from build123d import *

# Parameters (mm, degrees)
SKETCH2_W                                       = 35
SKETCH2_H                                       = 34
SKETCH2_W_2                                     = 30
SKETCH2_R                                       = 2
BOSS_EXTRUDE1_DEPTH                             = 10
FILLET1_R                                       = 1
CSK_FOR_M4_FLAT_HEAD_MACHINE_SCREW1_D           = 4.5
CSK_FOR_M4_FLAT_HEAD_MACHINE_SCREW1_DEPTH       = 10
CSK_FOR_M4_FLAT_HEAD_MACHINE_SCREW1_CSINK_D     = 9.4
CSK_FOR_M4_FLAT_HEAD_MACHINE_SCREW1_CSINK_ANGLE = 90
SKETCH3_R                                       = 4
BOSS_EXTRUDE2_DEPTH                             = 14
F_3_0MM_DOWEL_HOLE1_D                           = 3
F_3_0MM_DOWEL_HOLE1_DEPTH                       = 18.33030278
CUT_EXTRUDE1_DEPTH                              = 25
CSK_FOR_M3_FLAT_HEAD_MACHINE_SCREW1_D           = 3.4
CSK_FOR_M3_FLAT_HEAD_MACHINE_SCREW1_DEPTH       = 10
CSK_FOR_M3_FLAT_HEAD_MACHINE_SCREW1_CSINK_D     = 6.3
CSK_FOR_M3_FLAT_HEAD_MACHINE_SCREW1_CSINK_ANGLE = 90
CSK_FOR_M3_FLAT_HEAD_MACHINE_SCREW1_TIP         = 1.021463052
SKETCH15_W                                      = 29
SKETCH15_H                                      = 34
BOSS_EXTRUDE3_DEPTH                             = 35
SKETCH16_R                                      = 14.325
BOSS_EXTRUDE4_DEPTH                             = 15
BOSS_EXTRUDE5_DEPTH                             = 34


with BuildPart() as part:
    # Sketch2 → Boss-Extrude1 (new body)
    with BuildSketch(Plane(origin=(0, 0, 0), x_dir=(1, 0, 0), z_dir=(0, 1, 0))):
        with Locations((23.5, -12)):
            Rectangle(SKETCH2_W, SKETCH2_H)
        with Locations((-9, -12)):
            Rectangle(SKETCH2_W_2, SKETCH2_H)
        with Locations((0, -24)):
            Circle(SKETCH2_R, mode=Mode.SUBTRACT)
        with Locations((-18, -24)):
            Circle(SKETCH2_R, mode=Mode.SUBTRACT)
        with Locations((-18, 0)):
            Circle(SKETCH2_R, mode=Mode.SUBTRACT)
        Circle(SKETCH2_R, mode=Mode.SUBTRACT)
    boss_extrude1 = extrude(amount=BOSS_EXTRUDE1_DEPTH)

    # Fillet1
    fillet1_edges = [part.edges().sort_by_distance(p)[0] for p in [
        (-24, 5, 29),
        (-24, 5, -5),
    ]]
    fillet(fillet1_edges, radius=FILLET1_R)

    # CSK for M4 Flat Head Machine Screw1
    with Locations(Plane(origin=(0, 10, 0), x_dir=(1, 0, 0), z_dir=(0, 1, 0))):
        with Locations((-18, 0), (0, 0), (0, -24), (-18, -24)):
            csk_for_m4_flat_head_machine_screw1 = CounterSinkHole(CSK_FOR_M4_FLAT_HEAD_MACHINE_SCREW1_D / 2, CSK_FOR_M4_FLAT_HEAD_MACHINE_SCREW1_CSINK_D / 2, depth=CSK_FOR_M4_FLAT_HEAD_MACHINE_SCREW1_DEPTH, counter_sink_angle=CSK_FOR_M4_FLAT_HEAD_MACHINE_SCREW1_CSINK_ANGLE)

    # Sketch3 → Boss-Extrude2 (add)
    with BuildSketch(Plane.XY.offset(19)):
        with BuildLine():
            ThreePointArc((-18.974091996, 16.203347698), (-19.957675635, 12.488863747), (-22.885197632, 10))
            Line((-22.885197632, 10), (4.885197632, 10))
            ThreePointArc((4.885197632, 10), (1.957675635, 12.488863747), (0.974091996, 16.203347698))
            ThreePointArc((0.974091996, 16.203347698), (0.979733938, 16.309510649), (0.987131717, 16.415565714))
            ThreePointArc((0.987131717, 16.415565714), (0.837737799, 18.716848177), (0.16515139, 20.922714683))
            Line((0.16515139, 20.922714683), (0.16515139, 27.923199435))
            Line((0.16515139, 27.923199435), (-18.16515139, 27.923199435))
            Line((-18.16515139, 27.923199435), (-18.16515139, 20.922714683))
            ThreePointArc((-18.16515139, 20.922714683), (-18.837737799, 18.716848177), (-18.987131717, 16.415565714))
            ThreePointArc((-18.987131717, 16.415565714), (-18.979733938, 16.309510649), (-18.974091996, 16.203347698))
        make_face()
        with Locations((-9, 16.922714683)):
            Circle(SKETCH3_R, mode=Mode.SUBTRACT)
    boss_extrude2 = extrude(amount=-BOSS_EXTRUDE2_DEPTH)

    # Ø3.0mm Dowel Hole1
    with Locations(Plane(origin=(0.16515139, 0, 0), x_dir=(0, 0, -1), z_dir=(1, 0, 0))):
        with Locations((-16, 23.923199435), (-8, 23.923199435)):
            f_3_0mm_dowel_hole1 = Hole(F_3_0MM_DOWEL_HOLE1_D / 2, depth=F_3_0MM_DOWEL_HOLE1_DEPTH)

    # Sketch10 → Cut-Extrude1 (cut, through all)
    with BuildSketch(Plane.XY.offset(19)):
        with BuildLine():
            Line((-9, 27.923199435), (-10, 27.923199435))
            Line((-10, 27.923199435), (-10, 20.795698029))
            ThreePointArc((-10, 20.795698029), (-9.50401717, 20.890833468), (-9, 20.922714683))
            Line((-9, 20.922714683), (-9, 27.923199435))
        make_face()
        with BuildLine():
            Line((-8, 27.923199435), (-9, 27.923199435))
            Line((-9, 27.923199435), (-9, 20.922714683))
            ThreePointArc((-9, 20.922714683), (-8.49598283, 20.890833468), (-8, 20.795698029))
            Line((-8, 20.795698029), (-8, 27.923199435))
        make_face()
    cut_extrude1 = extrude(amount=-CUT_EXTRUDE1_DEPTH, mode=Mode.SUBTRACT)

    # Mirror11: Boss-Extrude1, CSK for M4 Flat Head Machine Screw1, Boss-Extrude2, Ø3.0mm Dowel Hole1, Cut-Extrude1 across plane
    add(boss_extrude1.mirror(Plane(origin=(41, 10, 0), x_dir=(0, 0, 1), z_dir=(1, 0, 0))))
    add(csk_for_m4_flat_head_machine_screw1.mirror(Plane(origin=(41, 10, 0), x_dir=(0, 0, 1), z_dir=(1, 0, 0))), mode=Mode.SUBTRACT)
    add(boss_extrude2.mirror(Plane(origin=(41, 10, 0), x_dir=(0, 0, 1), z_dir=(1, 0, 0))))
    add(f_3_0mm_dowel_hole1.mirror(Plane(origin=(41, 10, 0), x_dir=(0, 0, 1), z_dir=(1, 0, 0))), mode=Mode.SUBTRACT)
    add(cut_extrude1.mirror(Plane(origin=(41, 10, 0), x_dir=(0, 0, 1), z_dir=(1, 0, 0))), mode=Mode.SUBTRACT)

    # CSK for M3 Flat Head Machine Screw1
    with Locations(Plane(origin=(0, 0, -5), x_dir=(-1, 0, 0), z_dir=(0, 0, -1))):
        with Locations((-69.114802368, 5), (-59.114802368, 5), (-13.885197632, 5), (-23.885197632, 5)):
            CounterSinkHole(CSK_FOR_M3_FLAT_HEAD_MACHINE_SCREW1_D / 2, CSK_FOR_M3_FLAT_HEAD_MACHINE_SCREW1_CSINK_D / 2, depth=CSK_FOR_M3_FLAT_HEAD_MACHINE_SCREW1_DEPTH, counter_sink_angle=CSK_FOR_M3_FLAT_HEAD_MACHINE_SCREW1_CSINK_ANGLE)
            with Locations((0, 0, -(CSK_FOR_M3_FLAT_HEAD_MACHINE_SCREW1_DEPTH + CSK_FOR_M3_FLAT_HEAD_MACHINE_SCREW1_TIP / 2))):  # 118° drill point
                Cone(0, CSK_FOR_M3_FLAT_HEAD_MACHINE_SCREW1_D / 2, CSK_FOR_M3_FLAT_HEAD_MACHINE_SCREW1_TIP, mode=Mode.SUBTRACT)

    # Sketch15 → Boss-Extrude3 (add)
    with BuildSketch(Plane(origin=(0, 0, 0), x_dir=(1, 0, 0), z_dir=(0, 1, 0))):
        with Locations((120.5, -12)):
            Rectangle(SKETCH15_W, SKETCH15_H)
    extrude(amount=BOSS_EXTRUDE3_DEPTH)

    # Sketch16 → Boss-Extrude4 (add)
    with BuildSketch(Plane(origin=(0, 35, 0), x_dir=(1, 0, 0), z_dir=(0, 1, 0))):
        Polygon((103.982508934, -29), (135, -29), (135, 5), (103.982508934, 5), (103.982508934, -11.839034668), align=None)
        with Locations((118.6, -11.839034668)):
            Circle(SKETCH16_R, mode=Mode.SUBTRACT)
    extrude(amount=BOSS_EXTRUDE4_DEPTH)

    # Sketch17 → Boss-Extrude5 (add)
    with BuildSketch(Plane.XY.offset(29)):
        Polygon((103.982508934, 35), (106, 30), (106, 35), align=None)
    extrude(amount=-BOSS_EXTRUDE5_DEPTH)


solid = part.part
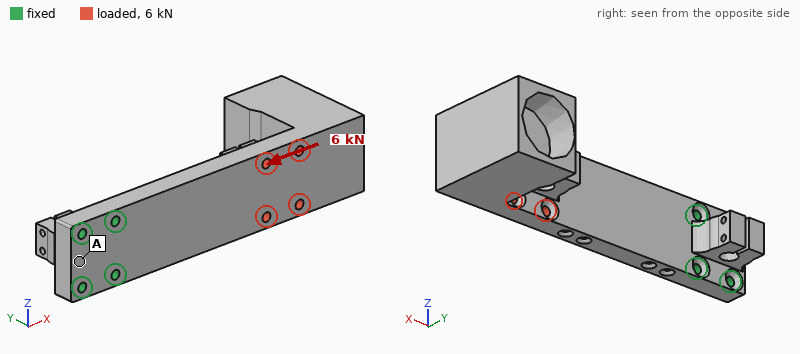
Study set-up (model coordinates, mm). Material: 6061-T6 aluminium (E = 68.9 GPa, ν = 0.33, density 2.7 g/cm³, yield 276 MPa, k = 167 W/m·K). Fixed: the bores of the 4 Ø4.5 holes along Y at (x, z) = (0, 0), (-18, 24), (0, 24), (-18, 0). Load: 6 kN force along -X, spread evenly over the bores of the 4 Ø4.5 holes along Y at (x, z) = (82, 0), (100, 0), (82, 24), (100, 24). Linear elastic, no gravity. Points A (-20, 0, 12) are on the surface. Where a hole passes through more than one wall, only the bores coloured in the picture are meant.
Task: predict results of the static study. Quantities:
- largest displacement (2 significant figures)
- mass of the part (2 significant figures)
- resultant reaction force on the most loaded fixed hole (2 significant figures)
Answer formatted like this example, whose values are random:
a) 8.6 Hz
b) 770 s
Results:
a) 0.33 mm
b) 240 g
c) 2.6 kN
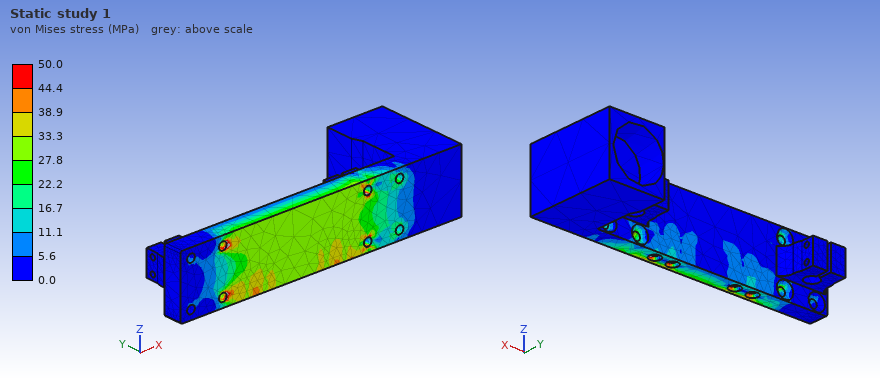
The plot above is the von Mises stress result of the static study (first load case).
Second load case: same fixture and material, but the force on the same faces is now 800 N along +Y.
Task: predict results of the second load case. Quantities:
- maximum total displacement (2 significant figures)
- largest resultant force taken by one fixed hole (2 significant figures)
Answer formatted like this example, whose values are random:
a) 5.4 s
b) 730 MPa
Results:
a) 2.0 mm
b) 1.5 kN
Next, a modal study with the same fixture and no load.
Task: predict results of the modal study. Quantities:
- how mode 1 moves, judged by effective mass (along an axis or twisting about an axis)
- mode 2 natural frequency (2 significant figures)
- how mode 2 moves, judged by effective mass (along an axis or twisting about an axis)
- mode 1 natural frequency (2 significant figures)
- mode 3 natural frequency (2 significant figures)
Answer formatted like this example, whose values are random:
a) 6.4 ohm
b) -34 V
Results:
a) along Y
b) 690 Hz
c) along Z
d) 240 Hz
e) 1500 Hz
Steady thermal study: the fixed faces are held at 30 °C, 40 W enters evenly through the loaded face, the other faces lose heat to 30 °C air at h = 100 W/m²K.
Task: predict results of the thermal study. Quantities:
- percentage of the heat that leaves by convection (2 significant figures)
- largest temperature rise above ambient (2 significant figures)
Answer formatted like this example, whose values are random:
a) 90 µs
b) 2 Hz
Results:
a) 73 %
b) 22 K
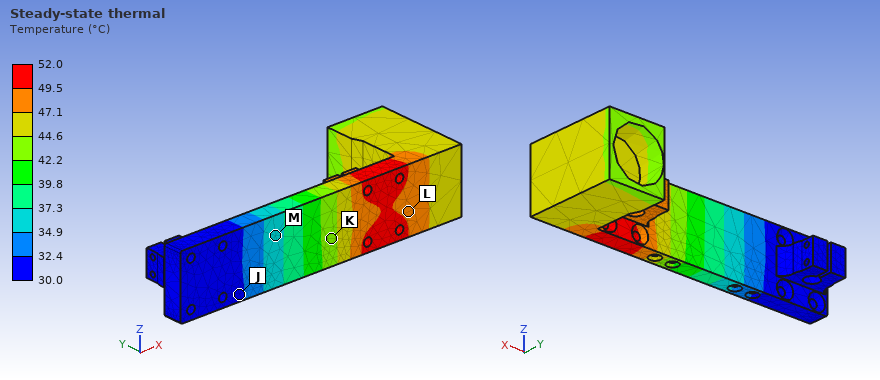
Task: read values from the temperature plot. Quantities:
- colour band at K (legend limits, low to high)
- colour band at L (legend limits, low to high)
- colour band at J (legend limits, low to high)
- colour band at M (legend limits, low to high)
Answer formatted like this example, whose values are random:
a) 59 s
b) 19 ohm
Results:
a) 42.2 to 44.6 °C
b) 47.1 to 49.5 °C
c) 30.0 to 32.4 °C
d) 34.9 to 37.3 °C
